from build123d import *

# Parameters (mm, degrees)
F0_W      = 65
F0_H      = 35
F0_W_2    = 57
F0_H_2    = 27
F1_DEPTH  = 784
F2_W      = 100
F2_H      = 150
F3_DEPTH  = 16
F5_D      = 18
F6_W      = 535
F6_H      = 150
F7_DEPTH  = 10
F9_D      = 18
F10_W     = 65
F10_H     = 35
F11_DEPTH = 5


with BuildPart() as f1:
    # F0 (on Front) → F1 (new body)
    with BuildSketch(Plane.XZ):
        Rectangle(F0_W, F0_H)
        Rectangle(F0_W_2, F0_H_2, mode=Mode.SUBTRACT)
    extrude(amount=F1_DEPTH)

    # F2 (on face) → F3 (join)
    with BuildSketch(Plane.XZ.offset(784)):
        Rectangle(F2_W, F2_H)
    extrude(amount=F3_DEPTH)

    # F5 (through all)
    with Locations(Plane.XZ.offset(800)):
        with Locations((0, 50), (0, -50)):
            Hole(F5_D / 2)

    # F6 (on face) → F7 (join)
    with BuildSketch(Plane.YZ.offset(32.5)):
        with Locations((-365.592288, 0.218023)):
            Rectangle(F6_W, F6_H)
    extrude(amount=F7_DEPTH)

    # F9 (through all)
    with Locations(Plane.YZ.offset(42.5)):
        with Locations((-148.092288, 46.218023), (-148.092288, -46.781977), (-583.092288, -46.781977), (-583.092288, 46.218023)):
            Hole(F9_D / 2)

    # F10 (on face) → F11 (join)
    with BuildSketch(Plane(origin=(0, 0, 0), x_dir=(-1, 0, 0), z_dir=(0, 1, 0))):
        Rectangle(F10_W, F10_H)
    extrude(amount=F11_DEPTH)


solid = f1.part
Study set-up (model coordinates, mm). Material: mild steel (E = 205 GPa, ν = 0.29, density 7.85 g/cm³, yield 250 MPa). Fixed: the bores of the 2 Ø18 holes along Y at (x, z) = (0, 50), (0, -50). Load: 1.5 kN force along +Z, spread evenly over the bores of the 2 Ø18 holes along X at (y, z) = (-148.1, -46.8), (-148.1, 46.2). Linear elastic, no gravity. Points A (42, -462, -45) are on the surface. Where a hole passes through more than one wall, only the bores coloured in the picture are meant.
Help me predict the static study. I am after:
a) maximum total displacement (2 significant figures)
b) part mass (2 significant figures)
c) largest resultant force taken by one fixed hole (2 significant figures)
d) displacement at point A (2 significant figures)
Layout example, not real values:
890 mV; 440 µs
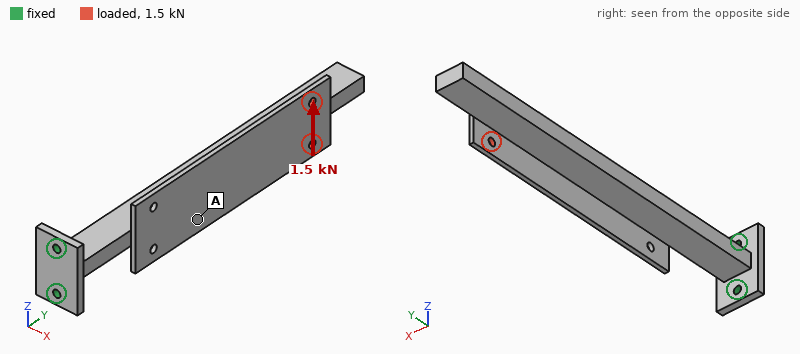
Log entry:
4.5 mm; 13 kg; 13 kN; 1.6 mm
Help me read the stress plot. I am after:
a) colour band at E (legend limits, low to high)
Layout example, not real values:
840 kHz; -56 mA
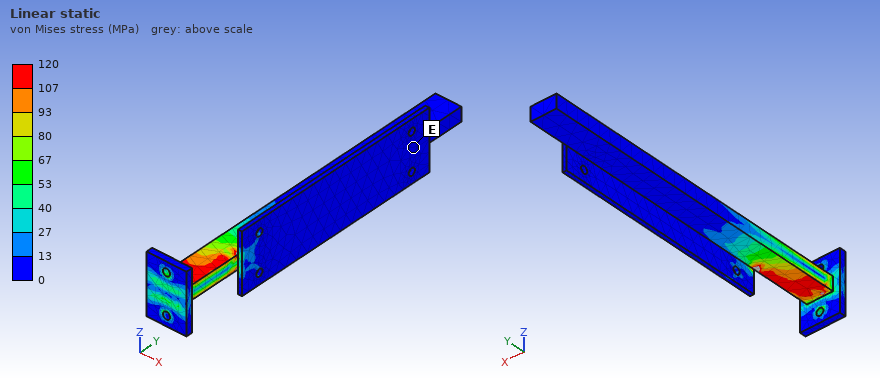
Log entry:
0 to 13 MPa
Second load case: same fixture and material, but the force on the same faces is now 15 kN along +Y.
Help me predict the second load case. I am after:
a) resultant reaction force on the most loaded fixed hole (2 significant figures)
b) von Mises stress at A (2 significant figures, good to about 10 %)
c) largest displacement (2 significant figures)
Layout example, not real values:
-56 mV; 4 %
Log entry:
7.6 kN; 9.7 MPa; 1.7 mm
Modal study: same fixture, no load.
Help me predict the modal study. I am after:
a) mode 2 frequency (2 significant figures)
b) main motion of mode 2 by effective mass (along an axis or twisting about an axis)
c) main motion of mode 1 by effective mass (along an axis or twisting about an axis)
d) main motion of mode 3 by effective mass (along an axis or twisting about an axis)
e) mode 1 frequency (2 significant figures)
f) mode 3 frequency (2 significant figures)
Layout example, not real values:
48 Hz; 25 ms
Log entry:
58 Hz; along X; along Z; twisting about Y; 46 Hz; 350 Hz
